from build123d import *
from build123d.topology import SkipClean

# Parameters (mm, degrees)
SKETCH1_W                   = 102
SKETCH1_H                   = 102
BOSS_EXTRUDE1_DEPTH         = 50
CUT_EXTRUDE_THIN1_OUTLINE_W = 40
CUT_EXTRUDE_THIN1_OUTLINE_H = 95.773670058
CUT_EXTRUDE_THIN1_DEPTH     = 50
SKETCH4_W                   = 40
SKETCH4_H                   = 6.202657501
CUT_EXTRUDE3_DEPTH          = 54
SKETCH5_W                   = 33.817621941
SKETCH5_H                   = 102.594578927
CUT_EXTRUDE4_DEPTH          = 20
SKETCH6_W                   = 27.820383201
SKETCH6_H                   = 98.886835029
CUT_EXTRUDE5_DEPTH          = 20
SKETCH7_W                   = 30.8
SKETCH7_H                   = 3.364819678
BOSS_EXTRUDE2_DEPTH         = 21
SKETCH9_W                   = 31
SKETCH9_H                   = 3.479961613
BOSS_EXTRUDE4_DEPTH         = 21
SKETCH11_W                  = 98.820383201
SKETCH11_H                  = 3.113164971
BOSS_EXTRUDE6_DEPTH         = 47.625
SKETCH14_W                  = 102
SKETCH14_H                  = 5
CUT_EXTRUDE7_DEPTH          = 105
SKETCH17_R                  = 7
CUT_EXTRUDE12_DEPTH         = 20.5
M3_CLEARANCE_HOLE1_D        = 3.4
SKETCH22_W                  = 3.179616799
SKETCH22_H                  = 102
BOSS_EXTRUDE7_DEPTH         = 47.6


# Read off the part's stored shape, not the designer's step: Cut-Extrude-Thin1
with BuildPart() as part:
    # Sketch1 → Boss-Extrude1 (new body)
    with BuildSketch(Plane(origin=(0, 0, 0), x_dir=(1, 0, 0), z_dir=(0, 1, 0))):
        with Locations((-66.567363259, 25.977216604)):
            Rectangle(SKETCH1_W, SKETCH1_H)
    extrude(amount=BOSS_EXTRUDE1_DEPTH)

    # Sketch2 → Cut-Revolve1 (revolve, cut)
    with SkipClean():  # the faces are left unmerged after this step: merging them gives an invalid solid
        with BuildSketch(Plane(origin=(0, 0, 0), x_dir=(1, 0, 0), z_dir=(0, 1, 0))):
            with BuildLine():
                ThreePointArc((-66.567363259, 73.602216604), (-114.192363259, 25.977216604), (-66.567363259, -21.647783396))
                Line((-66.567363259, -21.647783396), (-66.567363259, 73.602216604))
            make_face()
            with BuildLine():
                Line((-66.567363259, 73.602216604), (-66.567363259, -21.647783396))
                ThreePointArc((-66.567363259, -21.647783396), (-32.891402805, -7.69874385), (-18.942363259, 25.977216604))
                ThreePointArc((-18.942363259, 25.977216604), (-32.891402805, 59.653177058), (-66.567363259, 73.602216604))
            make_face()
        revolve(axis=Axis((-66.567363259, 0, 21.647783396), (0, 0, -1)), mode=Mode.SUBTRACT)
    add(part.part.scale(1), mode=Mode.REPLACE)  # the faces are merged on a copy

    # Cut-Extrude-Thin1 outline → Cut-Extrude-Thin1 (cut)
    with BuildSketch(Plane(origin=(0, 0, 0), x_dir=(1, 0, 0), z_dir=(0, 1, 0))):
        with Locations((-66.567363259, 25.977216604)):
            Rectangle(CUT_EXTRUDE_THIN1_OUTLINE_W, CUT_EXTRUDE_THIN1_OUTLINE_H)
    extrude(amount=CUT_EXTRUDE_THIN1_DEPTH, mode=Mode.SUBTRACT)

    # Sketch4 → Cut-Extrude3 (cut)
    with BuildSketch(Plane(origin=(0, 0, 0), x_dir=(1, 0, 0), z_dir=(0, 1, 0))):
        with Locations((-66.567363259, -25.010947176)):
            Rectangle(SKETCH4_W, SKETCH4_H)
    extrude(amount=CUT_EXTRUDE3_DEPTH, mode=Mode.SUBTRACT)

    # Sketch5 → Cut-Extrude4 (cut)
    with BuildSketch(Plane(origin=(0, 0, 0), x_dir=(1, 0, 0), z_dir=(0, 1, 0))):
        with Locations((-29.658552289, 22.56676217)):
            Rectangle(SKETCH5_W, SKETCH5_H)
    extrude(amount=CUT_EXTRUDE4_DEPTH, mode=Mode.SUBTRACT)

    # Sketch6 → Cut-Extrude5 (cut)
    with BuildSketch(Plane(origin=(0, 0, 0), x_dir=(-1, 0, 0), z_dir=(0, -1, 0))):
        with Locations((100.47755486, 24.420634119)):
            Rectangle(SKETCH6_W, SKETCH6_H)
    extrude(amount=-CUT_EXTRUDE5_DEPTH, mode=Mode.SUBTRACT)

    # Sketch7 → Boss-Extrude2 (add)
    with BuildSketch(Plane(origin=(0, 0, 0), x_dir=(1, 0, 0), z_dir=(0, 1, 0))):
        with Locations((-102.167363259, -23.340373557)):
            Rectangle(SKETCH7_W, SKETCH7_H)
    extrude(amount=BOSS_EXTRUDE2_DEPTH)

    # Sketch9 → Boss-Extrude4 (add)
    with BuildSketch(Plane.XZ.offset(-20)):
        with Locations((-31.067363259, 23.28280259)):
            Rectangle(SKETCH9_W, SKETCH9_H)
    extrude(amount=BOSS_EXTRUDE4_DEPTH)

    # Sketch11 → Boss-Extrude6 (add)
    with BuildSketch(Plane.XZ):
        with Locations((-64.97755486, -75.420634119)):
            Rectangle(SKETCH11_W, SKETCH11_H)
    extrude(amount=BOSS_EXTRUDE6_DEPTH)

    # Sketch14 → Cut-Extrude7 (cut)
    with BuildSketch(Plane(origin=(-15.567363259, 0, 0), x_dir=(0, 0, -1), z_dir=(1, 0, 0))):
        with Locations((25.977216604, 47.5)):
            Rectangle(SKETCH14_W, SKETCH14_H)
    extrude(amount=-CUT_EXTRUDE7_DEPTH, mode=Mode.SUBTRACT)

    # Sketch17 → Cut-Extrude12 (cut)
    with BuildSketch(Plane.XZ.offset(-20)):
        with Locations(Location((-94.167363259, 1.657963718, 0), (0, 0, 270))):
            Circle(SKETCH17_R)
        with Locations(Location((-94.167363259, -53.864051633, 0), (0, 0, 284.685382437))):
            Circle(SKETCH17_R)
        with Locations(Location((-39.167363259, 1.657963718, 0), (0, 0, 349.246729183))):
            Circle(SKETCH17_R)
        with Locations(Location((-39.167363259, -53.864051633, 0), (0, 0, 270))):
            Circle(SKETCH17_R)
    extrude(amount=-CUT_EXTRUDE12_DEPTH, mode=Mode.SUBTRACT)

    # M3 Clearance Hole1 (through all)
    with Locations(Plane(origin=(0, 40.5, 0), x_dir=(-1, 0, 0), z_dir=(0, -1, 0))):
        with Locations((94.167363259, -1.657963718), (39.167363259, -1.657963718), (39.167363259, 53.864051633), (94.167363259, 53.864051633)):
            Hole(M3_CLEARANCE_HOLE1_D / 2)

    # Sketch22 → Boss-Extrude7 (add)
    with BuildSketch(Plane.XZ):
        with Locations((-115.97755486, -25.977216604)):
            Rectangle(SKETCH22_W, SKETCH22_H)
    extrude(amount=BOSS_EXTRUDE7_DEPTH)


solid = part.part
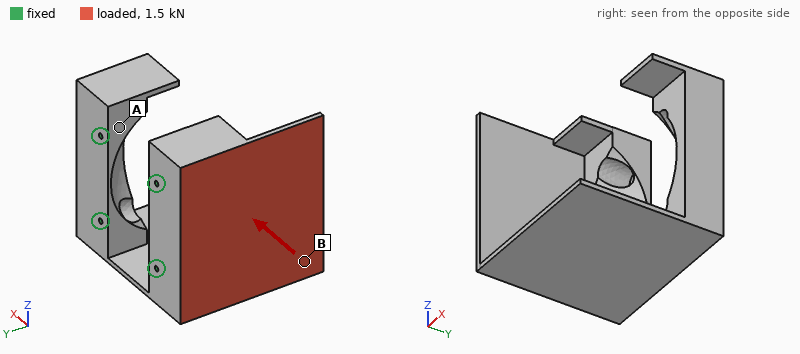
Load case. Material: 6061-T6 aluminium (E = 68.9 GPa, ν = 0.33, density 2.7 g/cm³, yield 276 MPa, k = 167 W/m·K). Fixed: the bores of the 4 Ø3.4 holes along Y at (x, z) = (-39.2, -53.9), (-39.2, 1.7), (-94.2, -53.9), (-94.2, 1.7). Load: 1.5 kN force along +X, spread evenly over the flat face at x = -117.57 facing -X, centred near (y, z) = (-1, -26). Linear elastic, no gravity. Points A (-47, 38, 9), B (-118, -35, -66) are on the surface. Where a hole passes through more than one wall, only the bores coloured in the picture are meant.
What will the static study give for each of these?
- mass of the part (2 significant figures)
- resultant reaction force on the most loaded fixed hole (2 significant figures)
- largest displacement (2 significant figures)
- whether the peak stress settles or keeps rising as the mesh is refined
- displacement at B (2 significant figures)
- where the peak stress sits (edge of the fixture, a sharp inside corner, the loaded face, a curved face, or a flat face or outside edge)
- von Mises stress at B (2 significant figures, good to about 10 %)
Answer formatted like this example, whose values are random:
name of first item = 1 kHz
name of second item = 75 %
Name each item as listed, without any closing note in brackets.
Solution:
mass of the part = 460 g
resultant reaction force on the most loaded fixed hole = 1.3 kN
largest displacement = 1.2 mm
whether the peak stress settles or keeps rising as the mesh is refined = keeps rising
displacement at B = 0.20 mm
where the peak stress sits = edge of the fixture
von Mises stress at B = 48 MPa
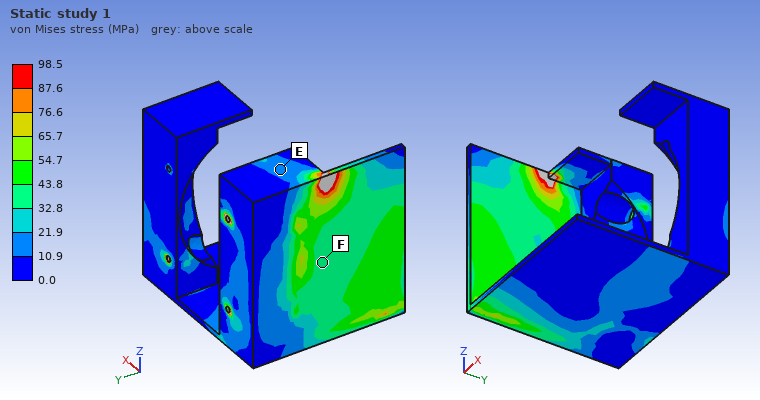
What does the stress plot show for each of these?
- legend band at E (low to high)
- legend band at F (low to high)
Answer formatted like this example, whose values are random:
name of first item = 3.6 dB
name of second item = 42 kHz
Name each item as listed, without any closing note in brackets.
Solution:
legend band at E = 10.9 to 21.9 MPa
legend band at F = 32.8 to 43.8 MPa
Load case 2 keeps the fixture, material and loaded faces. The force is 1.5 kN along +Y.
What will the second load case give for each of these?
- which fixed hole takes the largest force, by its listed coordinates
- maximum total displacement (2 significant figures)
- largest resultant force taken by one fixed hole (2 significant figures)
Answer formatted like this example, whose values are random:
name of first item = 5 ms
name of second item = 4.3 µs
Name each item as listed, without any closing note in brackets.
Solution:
which fixed hole takes the largest force, by its listed coordinates = (-94.2, -53.9)
maximum total displacement = 0.22 mm
largest resultant force taken by one fixed hole = 1.3 kN
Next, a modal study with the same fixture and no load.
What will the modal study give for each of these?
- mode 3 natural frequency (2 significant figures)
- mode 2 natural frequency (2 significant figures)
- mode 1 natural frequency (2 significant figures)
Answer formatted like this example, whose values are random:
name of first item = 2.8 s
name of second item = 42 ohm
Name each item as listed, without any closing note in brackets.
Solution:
mode 3 natural frequency = 1700 Hz
mode 2 natural frequency = 890 Hz
mode 1 natural frequency = 700 Hz
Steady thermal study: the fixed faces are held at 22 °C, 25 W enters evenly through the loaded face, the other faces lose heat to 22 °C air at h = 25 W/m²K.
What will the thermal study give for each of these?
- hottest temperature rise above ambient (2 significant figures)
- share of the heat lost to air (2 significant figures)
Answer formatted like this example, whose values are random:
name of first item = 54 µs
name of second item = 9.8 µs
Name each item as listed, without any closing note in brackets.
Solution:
hottest temperature rise above ambient = 14 K
share of the heat lost to air = 20 %
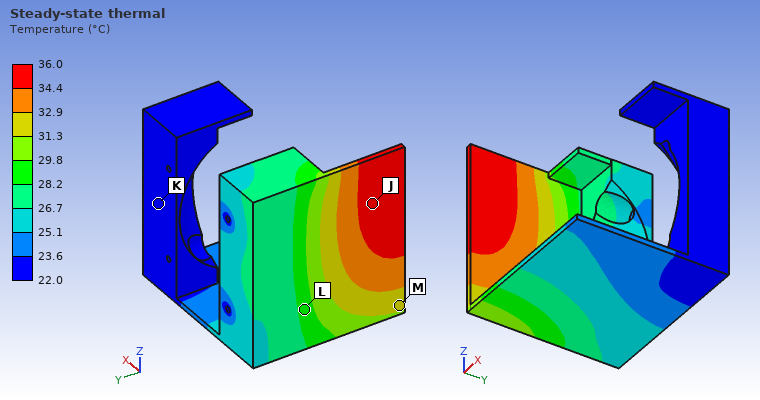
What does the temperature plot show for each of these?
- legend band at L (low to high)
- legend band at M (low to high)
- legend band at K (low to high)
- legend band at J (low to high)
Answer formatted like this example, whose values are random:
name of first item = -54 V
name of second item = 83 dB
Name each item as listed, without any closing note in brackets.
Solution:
legend band at L = 28.2 to 29.8 °C
legend band at M = 31.3 to 32.9 °C
legend band at K = 22.0 to 23.6 °C
legend band at J = 34.4 to 36.0 °C
